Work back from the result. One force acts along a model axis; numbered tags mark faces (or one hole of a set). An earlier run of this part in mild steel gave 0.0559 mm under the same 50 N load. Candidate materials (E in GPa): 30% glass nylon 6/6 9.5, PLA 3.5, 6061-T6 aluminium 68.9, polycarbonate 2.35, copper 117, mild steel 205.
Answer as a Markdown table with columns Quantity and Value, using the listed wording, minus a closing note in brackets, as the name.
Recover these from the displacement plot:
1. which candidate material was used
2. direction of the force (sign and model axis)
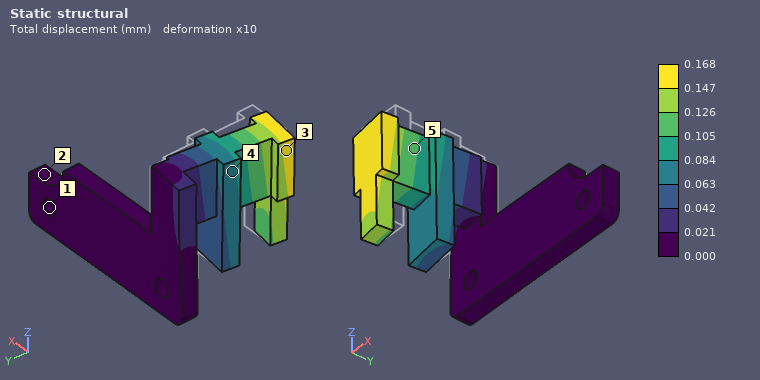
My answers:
| Quantity | Value |
|---|---|
| which candidate material was used | 6061-T6 aluminium |
| direction of the force | -X |
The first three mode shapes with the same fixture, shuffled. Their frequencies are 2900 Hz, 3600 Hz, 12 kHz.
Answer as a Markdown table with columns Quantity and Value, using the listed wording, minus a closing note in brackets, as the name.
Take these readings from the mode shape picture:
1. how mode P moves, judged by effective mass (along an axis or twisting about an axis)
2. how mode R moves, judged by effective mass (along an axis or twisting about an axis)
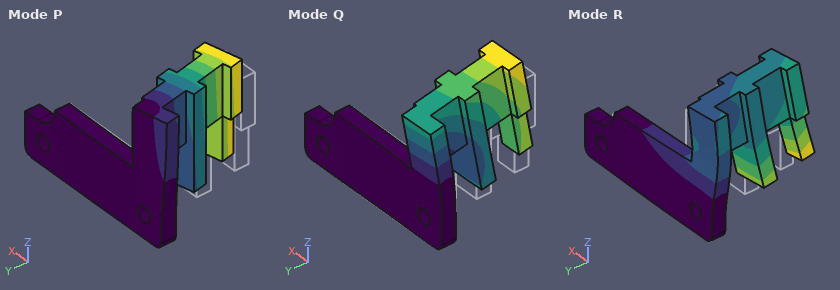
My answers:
| Quantity | Value |
|---|---|
| how mode P moves, judged by effective mass | along X |
| how mode R moves, judged by effective mass | along Y |
